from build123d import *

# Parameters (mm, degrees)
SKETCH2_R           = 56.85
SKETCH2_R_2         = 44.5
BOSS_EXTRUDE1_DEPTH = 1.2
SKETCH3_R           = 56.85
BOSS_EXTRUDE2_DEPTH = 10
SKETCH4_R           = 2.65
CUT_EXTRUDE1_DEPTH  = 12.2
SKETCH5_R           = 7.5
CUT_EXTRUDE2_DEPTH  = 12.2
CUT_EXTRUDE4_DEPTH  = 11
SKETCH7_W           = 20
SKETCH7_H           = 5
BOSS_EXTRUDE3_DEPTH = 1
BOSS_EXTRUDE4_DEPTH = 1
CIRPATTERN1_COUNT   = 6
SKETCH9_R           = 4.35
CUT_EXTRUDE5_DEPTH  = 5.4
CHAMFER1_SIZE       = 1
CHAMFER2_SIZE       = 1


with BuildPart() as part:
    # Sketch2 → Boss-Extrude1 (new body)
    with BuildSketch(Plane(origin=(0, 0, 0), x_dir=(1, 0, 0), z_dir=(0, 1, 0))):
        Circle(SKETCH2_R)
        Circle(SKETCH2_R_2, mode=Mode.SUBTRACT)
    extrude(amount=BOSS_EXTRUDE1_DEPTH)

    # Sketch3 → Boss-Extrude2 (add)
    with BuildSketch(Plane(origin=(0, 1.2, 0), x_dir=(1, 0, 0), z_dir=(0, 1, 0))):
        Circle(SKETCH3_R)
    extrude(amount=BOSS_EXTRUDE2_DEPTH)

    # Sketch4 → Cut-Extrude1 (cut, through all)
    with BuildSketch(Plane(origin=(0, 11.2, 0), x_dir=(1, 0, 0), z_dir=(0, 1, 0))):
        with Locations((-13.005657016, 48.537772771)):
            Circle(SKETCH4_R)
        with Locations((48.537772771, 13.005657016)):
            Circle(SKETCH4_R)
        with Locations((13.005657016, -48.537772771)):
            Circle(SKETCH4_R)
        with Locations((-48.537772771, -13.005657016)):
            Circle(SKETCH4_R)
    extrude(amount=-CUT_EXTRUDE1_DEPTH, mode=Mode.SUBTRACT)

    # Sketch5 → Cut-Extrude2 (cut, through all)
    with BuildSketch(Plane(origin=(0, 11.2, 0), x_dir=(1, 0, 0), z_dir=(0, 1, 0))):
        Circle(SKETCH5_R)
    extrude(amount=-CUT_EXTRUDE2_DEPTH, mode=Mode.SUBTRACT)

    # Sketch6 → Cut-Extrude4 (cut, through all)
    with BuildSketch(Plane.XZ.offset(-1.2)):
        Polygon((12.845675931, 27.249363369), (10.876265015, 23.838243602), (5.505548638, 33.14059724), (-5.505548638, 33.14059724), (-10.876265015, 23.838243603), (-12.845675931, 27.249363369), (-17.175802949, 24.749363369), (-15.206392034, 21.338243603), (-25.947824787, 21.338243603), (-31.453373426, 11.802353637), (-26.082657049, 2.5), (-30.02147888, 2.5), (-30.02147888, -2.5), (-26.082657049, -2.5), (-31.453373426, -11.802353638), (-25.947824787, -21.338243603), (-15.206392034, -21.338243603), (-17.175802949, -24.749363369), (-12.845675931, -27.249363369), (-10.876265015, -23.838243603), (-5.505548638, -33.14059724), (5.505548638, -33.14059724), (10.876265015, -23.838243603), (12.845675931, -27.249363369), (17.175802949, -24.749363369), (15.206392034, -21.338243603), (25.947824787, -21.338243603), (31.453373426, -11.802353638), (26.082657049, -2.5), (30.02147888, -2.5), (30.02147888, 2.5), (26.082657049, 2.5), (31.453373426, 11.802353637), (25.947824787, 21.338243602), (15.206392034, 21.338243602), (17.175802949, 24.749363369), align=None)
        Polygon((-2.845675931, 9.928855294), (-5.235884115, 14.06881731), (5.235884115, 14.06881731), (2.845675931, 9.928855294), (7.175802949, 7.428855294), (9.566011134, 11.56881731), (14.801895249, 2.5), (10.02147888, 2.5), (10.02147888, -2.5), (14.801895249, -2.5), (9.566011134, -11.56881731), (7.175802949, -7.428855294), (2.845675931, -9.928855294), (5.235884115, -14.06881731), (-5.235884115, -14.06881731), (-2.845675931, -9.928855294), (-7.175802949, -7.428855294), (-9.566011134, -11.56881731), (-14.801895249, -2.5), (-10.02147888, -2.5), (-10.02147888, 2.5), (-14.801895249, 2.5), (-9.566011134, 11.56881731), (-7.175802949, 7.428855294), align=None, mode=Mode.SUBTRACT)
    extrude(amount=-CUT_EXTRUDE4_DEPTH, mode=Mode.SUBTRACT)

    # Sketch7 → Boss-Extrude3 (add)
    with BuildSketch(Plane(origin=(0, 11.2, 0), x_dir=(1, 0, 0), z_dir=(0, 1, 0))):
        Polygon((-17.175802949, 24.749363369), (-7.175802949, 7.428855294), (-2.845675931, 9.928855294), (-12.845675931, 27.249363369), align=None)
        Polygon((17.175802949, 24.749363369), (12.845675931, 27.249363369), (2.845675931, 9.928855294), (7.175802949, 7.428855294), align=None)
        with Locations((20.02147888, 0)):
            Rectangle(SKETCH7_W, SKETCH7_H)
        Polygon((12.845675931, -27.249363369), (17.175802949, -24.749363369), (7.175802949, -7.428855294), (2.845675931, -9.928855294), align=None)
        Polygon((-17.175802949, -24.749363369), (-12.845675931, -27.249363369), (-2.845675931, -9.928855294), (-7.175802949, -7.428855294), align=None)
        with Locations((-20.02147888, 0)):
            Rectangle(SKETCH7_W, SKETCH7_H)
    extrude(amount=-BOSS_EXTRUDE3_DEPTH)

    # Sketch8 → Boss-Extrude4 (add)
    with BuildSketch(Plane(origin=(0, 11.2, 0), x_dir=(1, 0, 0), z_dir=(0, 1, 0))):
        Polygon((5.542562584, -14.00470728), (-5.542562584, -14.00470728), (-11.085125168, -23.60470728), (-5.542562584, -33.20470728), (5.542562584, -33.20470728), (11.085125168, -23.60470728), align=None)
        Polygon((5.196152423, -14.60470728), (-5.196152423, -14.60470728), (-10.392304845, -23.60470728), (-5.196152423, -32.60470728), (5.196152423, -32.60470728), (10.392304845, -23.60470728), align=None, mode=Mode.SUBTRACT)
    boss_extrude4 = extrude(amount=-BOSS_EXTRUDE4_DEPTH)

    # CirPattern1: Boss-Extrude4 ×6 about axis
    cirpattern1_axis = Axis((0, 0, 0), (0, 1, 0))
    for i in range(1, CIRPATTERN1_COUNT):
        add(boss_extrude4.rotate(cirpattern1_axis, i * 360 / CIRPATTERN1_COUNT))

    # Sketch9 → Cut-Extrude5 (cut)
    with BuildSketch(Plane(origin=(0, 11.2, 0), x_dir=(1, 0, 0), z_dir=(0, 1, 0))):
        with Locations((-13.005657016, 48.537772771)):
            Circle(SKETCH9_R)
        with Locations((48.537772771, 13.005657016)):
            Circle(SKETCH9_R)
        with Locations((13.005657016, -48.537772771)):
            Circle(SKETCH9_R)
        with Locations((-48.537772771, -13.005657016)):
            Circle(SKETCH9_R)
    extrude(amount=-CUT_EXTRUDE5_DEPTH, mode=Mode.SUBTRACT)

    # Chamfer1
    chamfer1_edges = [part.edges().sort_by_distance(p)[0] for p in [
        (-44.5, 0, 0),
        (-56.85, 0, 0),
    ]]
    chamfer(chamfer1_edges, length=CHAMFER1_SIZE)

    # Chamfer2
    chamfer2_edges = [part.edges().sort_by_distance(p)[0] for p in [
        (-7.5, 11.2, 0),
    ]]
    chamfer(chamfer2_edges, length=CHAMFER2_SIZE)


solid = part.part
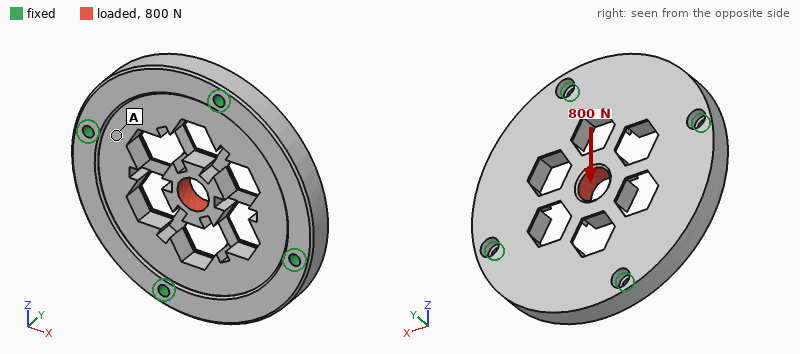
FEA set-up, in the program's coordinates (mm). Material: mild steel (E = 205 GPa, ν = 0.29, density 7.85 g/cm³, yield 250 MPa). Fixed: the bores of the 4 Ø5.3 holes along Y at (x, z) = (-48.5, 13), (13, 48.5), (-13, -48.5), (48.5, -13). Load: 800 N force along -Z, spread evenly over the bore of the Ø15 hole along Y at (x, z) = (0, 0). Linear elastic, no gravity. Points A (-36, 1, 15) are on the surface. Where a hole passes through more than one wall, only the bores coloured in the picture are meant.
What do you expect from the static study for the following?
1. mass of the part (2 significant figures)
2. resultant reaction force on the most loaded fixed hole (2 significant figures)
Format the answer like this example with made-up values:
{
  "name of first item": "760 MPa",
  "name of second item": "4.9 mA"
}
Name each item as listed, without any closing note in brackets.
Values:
{
  "mass of the part": "620 g",
  "resultant reaction force on the most loaded fixed hole": "230 N"
}
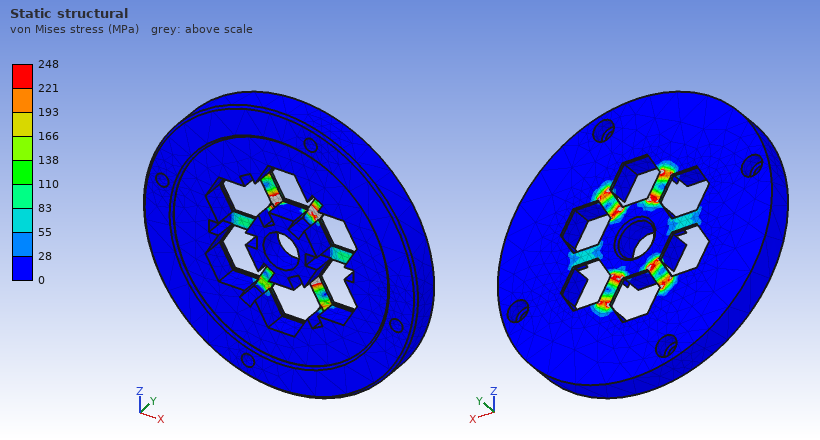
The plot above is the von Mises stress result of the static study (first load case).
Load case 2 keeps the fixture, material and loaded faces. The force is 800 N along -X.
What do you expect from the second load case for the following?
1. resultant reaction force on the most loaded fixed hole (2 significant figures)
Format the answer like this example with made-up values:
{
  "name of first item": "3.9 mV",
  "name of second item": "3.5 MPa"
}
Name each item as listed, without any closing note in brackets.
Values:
{
  "resultant reaction force on the most loaded fixed hole": "230 N"
}
